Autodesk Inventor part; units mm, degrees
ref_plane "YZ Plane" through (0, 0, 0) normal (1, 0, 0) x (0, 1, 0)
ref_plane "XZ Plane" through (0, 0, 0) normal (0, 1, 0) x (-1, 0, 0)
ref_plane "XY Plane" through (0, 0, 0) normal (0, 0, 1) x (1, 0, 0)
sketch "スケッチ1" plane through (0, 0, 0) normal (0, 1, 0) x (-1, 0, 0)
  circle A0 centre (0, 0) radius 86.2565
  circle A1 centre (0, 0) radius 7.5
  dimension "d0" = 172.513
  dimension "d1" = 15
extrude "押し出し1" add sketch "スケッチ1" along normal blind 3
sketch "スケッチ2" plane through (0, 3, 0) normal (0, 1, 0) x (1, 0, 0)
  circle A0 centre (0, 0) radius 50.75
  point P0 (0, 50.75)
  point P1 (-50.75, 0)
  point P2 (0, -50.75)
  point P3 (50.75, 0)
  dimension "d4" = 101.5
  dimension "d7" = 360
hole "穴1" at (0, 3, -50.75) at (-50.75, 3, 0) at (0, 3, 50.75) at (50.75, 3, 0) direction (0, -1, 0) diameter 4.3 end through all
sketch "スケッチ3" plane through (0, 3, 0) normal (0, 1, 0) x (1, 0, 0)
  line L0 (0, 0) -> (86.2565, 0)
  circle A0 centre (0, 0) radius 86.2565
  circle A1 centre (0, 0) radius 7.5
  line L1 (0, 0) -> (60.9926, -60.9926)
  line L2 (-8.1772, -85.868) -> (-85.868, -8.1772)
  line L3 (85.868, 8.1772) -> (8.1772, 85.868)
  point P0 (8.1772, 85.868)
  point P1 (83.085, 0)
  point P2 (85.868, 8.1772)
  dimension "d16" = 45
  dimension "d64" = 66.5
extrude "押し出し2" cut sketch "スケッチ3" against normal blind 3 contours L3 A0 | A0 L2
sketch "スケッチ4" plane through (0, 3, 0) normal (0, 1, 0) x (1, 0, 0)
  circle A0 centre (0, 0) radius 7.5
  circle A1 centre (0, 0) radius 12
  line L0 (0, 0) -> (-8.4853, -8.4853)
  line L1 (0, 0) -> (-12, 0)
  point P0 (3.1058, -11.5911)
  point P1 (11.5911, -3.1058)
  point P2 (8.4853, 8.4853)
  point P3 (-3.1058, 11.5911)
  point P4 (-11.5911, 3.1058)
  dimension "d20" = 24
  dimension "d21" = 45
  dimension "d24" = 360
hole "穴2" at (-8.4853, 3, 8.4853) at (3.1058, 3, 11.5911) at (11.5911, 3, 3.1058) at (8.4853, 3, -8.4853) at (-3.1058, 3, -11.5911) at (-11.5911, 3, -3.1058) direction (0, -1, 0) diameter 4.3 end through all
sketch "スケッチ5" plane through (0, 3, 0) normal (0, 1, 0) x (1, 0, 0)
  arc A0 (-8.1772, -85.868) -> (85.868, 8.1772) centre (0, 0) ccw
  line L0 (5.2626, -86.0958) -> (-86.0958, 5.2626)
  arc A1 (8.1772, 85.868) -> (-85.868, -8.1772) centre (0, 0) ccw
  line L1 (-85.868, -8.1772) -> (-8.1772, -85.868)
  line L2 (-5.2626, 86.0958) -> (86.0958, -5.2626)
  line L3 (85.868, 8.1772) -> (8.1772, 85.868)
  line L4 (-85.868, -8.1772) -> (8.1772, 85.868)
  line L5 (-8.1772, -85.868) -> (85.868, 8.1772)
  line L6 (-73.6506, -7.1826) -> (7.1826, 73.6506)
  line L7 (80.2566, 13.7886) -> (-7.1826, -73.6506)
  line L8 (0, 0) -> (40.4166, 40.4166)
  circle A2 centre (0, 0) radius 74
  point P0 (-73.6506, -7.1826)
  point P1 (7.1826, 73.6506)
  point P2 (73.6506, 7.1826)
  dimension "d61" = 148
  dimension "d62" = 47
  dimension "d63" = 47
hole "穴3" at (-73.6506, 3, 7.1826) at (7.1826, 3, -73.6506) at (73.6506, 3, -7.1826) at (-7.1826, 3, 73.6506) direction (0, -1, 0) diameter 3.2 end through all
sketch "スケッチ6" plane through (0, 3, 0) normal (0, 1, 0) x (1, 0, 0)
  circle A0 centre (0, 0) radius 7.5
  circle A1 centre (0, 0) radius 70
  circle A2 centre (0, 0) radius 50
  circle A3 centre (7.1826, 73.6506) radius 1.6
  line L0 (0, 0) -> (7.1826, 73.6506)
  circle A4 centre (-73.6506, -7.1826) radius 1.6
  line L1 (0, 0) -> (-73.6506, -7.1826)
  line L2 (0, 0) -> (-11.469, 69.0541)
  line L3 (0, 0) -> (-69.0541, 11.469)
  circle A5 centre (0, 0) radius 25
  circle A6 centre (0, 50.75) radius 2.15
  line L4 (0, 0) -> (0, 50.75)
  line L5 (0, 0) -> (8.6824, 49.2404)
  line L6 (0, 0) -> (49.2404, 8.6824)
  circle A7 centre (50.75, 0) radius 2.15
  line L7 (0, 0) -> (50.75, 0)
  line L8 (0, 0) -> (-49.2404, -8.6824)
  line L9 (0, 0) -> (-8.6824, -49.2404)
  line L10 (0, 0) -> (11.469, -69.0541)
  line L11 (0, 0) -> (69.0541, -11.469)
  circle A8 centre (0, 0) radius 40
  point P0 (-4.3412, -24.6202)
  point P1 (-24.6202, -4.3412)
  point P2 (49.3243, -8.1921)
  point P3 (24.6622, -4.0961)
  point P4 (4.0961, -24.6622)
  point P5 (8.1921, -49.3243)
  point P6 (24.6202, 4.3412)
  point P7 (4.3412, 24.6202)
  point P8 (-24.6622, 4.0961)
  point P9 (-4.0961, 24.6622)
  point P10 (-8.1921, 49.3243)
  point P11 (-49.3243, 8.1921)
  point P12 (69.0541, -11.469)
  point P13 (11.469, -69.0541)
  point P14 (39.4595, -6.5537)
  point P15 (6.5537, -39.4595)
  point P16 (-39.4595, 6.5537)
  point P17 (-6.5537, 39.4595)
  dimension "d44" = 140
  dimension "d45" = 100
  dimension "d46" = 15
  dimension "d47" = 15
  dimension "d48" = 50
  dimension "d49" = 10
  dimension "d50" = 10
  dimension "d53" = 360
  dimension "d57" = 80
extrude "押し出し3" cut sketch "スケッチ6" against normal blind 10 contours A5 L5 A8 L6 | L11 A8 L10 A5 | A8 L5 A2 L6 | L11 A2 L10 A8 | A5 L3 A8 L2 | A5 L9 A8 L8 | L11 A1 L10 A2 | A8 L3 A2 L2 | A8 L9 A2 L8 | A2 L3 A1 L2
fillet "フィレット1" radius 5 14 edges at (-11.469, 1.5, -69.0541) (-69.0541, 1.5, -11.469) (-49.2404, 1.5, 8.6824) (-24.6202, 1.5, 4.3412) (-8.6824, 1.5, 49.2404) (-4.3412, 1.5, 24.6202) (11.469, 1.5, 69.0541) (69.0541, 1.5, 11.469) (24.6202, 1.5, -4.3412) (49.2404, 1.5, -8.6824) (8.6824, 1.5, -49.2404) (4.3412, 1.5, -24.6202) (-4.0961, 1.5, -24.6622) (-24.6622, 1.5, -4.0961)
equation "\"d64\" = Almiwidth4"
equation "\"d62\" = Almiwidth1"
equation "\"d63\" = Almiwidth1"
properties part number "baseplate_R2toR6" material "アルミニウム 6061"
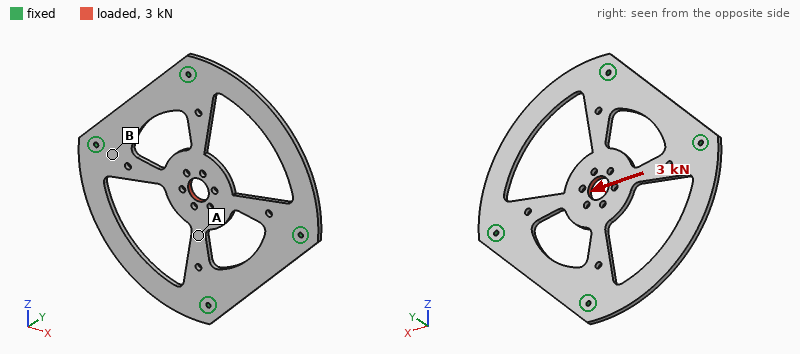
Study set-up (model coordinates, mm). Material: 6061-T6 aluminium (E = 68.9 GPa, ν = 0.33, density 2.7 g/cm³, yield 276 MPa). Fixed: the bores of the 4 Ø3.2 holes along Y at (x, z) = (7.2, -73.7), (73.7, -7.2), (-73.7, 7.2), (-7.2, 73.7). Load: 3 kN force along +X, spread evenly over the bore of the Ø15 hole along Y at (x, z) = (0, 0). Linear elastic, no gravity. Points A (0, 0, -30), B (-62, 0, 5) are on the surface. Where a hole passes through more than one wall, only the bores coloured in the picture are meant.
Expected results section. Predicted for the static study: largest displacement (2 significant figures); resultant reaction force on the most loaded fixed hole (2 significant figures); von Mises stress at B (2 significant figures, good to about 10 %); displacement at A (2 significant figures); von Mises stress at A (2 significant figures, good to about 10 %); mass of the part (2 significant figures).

36 µm
1.3 kN
24 MPa
22 µm
12 MPa
100 g
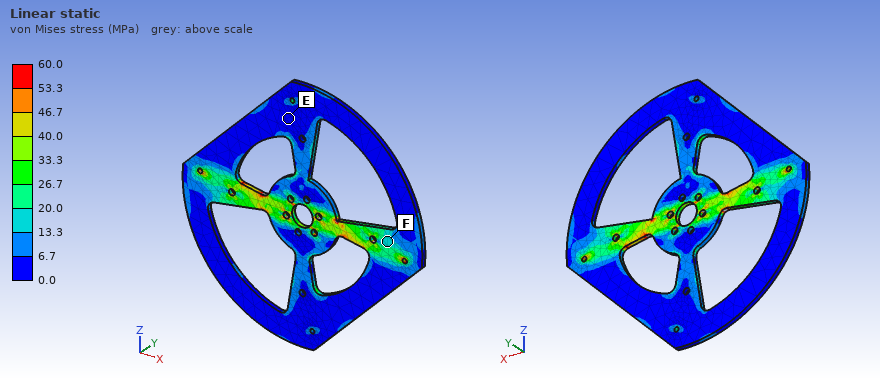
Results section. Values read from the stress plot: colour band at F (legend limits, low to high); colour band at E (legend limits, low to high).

13.3 to 20.0 MPa
0.0 to 6.7 MPa
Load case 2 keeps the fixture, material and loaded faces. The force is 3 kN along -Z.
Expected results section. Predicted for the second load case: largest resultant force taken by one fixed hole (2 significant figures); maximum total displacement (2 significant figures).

1.3 kN
36 µm
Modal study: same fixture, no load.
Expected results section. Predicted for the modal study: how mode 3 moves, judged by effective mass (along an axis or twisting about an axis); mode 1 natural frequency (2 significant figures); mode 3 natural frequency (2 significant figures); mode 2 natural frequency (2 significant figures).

along Y
850 Hz
920 Hz
860 Hz
